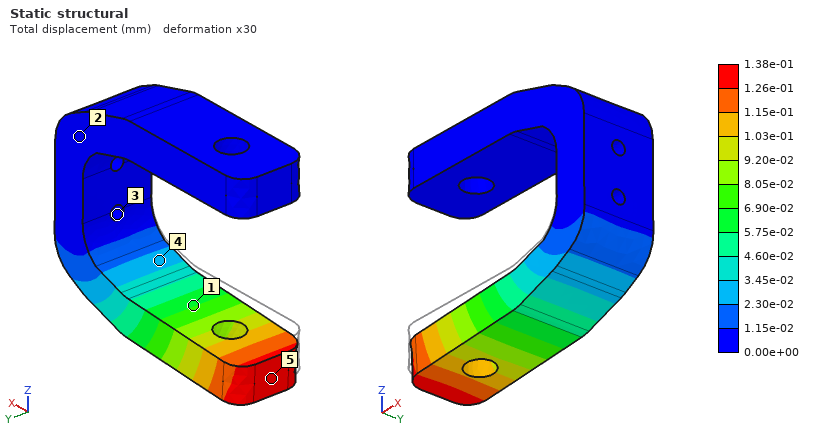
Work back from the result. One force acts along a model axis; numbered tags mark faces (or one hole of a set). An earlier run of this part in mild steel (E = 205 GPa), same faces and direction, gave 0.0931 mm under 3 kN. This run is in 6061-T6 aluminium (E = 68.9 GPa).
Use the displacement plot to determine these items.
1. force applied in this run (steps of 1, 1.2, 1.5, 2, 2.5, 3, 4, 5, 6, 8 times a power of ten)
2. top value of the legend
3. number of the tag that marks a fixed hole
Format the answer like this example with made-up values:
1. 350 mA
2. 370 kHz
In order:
1. 1.5 kN
2. 1.38e-01 mm
3. 3
